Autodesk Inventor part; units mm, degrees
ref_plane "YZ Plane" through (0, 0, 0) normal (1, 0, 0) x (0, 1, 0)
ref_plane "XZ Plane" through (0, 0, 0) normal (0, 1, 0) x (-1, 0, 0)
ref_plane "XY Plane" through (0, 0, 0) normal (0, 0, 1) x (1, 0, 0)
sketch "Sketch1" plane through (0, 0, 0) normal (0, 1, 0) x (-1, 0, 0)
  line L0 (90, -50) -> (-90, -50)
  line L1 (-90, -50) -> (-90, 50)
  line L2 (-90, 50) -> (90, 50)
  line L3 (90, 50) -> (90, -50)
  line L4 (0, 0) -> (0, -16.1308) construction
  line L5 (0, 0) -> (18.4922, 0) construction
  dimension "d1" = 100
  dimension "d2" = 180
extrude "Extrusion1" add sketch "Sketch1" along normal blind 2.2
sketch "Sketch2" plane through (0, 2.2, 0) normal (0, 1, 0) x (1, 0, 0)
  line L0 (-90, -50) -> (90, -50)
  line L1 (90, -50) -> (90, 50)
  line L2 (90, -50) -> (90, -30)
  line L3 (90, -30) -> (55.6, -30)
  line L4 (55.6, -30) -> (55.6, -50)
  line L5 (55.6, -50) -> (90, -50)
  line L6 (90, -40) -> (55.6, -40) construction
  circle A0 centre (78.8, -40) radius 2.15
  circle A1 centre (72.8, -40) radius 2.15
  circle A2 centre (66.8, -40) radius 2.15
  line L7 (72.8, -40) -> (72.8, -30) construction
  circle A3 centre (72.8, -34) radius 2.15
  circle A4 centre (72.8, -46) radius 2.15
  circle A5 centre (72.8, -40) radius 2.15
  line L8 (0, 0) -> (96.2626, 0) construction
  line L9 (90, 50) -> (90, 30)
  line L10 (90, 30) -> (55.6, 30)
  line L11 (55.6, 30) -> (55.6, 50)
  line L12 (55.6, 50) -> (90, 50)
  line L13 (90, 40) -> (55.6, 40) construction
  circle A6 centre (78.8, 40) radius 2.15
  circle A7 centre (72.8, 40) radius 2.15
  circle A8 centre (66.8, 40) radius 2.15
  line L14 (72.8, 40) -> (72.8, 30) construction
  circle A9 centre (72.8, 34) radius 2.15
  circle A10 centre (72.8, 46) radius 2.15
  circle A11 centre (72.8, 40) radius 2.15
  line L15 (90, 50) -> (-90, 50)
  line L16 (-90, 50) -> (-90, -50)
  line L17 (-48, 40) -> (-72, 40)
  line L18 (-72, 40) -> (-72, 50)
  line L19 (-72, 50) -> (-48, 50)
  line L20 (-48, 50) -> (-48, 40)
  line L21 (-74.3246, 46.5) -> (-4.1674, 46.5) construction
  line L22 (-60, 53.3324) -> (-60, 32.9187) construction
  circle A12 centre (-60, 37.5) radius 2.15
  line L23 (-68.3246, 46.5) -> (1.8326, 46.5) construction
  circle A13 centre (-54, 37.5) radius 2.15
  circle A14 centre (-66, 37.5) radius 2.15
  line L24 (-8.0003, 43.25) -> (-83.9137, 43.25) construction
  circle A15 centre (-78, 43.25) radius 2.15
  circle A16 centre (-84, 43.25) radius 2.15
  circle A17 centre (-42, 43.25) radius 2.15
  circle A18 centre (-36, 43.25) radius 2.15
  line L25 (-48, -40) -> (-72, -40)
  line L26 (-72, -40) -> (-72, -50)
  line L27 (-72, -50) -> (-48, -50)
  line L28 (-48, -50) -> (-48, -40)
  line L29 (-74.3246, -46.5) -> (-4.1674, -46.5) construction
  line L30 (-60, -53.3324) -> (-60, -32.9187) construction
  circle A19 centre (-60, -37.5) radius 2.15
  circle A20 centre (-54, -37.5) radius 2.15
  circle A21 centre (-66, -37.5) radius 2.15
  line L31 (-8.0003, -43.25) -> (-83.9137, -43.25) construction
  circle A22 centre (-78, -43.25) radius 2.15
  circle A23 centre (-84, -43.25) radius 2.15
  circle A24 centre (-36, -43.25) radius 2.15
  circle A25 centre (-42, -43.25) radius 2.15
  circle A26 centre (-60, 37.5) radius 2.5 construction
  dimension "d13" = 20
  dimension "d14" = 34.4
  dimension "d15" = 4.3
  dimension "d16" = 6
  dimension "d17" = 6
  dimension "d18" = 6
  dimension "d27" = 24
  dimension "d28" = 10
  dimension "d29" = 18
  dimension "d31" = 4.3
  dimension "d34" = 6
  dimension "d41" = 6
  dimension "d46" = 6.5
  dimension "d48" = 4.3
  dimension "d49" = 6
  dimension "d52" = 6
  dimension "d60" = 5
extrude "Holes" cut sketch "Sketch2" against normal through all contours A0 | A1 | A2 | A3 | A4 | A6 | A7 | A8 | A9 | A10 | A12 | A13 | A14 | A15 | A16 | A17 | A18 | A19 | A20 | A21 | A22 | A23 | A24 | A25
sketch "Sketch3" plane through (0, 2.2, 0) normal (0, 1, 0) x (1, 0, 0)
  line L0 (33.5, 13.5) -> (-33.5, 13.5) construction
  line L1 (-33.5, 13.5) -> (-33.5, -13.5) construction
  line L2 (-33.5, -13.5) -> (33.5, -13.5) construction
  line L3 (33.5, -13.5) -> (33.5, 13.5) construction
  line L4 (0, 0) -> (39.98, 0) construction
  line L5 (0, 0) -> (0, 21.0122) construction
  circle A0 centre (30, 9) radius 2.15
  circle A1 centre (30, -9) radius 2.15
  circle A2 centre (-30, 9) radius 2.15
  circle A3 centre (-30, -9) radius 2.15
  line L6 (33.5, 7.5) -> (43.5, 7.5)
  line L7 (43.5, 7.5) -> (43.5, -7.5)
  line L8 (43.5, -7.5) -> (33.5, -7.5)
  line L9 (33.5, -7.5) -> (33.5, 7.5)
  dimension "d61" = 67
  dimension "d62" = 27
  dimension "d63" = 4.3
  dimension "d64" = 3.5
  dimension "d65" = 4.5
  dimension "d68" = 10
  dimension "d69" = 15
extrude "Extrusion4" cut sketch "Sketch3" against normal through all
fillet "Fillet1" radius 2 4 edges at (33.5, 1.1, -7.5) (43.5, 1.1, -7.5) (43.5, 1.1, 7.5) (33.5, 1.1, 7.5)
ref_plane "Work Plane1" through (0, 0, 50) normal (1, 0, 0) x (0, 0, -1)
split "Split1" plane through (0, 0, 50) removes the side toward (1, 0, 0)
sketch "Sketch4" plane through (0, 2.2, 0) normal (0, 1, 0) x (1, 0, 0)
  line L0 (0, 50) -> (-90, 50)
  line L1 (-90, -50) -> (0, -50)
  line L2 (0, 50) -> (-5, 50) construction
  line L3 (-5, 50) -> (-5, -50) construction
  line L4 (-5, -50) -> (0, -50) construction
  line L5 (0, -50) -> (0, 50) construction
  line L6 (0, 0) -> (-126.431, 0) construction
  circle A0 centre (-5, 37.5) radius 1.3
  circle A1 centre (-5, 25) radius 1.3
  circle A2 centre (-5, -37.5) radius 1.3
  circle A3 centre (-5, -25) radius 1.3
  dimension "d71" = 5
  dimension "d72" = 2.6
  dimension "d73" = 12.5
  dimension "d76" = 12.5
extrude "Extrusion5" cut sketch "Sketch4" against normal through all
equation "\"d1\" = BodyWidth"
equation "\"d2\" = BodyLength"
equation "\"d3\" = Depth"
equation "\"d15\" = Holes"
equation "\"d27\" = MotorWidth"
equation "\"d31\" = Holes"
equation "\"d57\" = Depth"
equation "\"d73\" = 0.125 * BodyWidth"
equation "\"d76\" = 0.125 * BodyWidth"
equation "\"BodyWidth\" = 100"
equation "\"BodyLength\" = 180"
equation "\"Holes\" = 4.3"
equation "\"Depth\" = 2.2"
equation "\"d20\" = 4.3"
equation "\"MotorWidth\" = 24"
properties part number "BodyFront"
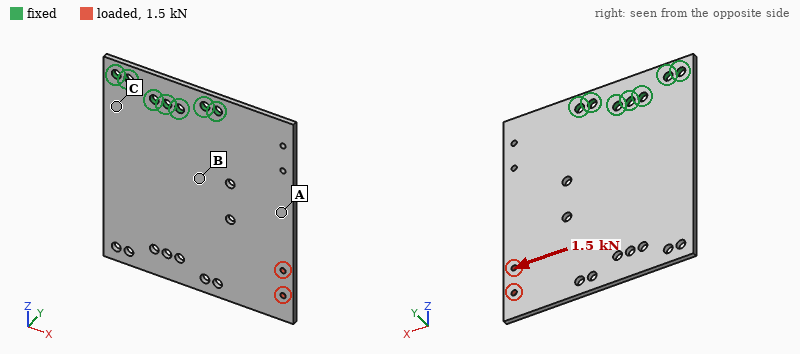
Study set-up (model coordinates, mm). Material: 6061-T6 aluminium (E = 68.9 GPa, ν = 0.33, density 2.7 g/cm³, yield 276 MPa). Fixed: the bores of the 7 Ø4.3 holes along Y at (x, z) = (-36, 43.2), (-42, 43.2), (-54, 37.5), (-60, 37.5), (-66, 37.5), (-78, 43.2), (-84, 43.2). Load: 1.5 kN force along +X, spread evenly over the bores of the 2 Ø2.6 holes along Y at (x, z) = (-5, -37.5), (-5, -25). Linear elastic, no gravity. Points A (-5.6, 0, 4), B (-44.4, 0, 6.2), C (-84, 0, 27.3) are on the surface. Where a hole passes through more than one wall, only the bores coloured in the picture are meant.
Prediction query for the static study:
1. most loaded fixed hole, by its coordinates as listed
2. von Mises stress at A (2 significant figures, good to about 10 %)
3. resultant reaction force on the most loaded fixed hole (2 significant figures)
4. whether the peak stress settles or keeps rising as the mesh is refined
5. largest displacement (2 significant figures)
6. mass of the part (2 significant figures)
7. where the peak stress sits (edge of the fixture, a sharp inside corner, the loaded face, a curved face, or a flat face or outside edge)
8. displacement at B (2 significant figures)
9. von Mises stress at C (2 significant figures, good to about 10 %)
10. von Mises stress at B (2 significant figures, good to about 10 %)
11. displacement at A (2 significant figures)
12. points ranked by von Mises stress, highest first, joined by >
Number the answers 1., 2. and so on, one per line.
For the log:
1. (-36, 43.2)
2. 11 MPa
3. 1.8 kN
4. keeps rising
5. 0.13 mm
6. 52 g
7. edge of the fixture
8. 0.039 mm
9. 45 MPa
10. 26 MPa
11. 0.070 mm
12. C > B > A
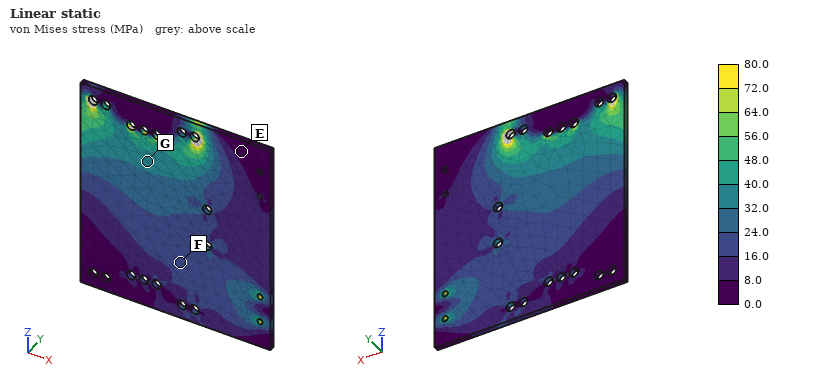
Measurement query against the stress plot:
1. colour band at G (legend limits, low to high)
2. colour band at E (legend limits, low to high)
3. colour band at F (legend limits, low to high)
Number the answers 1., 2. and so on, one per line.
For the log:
1. 32.0 to 40.0 MPa
2. 0.0 to 8.0 MPa
3. 16.0 to 24.0 MPa
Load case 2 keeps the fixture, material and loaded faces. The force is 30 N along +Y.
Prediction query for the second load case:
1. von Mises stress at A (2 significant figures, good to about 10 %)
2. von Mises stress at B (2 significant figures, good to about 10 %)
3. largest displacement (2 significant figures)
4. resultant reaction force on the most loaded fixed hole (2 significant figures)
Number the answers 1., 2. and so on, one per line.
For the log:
1. 19 MPa
2. 19 MPa
3. 1.5 mm
4. 37 N
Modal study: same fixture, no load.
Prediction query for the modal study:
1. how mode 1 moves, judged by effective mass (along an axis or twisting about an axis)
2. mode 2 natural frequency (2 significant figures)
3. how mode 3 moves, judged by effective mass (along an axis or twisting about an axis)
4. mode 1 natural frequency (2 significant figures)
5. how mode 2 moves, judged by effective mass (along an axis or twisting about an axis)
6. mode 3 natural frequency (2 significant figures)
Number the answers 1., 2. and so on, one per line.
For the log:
1. along Y
2. 480 Hz
3. along Y
4. 220 Hz
5. twisting about Z
6. 1100 Hz
